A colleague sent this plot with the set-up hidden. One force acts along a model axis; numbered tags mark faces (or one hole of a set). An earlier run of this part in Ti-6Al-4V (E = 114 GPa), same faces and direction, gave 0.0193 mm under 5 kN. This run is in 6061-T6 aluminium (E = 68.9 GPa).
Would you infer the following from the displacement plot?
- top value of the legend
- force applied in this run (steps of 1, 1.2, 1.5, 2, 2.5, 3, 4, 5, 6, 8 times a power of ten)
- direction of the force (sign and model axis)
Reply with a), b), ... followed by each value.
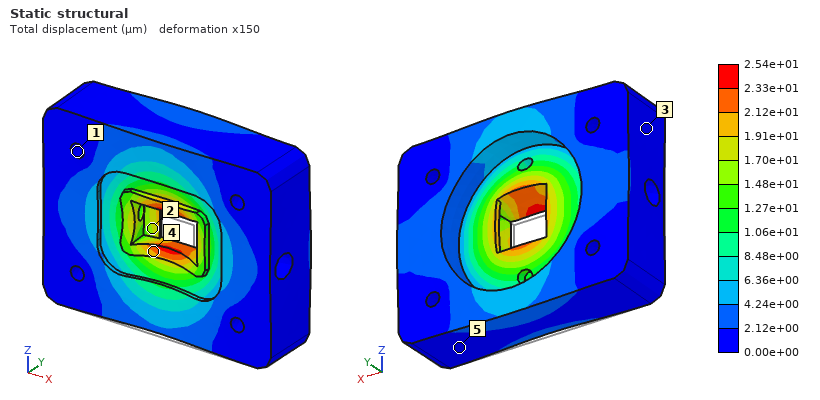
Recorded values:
a) 2.54e+01 µm
b) 4 kN
c) +Y
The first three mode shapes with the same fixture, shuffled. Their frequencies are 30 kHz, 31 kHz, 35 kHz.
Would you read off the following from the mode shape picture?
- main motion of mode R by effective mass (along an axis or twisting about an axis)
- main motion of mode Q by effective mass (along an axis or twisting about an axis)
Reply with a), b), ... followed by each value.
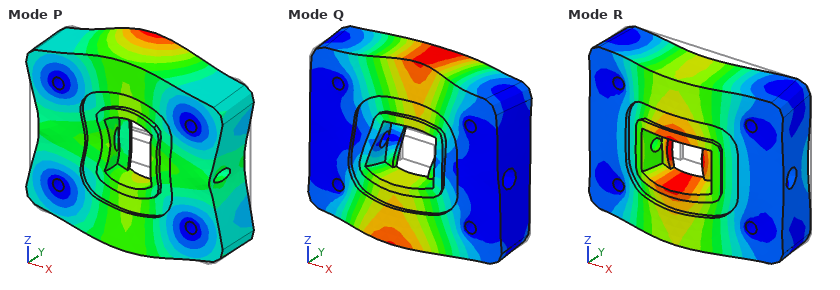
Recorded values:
a) along Y
b) twisting about X
